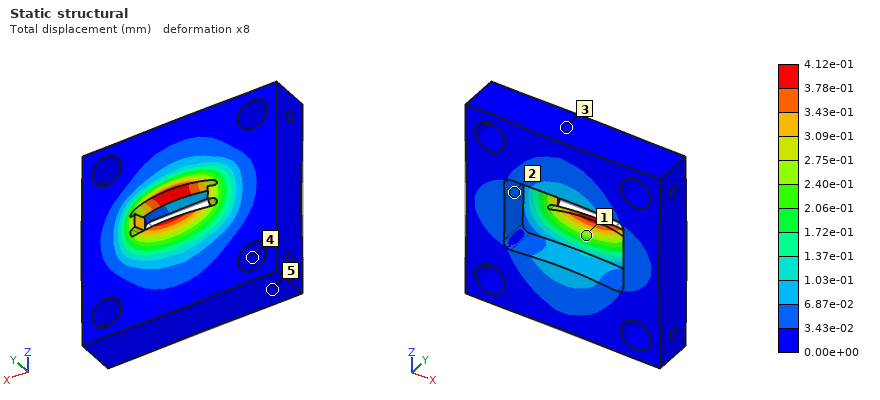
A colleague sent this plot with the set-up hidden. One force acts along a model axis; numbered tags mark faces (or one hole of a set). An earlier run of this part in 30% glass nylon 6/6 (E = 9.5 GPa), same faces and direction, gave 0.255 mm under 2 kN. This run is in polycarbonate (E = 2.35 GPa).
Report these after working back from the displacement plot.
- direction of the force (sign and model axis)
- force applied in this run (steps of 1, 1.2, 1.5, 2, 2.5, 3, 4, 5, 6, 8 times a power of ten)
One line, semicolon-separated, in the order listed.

+Y; 800 N
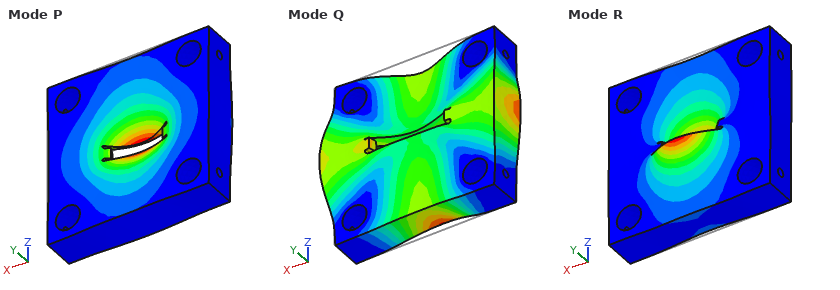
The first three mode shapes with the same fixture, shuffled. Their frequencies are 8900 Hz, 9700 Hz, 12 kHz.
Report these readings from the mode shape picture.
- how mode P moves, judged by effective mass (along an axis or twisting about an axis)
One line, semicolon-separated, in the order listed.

along Y
